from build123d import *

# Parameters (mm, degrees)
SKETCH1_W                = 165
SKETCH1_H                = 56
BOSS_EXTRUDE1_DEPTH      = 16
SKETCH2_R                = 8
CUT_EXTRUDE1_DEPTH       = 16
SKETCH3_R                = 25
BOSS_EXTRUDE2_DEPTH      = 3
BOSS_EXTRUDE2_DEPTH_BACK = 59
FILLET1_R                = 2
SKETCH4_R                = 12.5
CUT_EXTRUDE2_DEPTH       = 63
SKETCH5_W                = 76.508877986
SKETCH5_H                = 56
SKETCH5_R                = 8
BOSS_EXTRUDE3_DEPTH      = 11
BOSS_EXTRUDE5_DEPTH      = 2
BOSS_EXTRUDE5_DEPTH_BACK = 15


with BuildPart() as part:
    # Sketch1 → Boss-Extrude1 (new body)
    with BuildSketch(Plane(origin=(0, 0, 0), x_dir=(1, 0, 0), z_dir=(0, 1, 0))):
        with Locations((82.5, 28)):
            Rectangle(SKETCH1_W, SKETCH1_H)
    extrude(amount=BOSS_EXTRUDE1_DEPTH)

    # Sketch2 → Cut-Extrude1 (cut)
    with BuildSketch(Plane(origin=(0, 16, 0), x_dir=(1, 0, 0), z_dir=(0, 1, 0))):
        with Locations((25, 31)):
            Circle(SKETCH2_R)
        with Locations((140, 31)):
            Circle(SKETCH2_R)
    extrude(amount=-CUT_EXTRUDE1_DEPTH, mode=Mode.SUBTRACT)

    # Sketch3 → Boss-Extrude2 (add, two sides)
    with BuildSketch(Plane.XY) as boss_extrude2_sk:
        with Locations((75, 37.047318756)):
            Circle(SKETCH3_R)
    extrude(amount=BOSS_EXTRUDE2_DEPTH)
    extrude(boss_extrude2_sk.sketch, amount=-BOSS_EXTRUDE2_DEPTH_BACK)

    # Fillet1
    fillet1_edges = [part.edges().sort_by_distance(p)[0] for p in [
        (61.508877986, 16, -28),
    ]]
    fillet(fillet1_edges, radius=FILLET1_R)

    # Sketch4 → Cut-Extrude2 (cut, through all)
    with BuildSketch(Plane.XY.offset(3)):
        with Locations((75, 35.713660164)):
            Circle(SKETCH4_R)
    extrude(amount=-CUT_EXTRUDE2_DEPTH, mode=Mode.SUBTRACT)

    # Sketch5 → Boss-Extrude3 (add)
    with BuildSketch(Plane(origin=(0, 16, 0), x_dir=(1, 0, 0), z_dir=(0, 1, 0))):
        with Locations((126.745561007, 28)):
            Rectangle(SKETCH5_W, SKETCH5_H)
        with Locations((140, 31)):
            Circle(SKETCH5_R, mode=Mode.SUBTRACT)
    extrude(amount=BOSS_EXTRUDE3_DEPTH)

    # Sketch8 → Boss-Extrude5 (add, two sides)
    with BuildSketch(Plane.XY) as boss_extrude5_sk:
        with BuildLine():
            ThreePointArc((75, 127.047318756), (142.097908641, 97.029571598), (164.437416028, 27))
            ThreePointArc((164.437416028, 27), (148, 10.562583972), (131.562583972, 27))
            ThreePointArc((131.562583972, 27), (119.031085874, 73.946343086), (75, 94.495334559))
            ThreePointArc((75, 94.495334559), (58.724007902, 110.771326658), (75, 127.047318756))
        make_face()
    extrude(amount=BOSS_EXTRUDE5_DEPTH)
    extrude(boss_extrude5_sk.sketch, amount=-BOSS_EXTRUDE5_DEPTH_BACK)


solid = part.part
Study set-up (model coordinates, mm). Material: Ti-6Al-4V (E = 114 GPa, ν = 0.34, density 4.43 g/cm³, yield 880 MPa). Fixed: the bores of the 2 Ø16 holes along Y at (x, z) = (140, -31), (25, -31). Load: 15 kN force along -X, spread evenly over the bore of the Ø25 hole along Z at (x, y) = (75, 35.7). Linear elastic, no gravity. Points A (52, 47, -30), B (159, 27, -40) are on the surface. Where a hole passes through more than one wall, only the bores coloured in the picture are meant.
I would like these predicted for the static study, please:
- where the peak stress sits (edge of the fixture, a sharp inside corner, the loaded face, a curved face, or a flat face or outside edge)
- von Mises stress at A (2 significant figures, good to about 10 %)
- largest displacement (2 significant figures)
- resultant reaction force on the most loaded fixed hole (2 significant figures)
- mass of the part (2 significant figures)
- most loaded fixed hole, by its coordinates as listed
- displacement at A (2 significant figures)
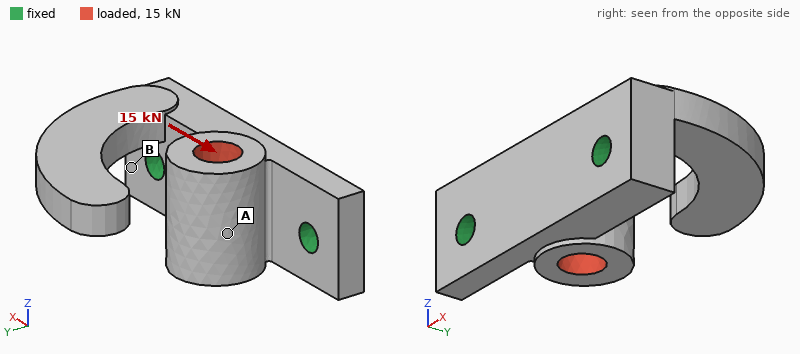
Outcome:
a curved face
10 MPa
28 µm
11 kN
1.5 kg
(140, -31)
26 µm
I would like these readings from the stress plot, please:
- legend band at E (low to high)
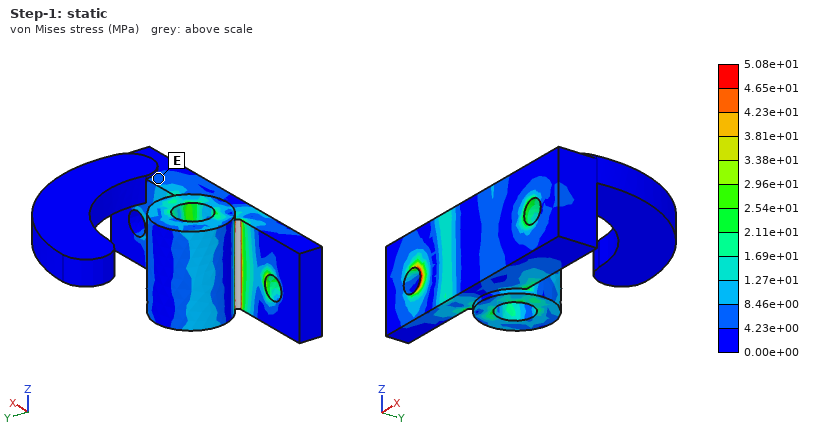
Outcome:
4.23e+00 to 8.46e+00 MPa
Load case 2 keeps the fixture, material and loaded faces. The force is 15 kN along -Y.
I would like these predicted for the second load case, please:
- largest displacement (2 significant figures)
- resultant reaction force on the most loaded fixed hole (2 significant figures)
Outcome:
30 µm
7.9 kN
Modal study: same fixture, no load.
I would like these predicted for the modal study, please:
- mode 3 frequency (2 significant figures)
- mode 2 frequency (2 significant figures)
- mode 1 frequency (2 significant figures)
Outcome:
2500 Hz
1100 Hz
690 Hz
